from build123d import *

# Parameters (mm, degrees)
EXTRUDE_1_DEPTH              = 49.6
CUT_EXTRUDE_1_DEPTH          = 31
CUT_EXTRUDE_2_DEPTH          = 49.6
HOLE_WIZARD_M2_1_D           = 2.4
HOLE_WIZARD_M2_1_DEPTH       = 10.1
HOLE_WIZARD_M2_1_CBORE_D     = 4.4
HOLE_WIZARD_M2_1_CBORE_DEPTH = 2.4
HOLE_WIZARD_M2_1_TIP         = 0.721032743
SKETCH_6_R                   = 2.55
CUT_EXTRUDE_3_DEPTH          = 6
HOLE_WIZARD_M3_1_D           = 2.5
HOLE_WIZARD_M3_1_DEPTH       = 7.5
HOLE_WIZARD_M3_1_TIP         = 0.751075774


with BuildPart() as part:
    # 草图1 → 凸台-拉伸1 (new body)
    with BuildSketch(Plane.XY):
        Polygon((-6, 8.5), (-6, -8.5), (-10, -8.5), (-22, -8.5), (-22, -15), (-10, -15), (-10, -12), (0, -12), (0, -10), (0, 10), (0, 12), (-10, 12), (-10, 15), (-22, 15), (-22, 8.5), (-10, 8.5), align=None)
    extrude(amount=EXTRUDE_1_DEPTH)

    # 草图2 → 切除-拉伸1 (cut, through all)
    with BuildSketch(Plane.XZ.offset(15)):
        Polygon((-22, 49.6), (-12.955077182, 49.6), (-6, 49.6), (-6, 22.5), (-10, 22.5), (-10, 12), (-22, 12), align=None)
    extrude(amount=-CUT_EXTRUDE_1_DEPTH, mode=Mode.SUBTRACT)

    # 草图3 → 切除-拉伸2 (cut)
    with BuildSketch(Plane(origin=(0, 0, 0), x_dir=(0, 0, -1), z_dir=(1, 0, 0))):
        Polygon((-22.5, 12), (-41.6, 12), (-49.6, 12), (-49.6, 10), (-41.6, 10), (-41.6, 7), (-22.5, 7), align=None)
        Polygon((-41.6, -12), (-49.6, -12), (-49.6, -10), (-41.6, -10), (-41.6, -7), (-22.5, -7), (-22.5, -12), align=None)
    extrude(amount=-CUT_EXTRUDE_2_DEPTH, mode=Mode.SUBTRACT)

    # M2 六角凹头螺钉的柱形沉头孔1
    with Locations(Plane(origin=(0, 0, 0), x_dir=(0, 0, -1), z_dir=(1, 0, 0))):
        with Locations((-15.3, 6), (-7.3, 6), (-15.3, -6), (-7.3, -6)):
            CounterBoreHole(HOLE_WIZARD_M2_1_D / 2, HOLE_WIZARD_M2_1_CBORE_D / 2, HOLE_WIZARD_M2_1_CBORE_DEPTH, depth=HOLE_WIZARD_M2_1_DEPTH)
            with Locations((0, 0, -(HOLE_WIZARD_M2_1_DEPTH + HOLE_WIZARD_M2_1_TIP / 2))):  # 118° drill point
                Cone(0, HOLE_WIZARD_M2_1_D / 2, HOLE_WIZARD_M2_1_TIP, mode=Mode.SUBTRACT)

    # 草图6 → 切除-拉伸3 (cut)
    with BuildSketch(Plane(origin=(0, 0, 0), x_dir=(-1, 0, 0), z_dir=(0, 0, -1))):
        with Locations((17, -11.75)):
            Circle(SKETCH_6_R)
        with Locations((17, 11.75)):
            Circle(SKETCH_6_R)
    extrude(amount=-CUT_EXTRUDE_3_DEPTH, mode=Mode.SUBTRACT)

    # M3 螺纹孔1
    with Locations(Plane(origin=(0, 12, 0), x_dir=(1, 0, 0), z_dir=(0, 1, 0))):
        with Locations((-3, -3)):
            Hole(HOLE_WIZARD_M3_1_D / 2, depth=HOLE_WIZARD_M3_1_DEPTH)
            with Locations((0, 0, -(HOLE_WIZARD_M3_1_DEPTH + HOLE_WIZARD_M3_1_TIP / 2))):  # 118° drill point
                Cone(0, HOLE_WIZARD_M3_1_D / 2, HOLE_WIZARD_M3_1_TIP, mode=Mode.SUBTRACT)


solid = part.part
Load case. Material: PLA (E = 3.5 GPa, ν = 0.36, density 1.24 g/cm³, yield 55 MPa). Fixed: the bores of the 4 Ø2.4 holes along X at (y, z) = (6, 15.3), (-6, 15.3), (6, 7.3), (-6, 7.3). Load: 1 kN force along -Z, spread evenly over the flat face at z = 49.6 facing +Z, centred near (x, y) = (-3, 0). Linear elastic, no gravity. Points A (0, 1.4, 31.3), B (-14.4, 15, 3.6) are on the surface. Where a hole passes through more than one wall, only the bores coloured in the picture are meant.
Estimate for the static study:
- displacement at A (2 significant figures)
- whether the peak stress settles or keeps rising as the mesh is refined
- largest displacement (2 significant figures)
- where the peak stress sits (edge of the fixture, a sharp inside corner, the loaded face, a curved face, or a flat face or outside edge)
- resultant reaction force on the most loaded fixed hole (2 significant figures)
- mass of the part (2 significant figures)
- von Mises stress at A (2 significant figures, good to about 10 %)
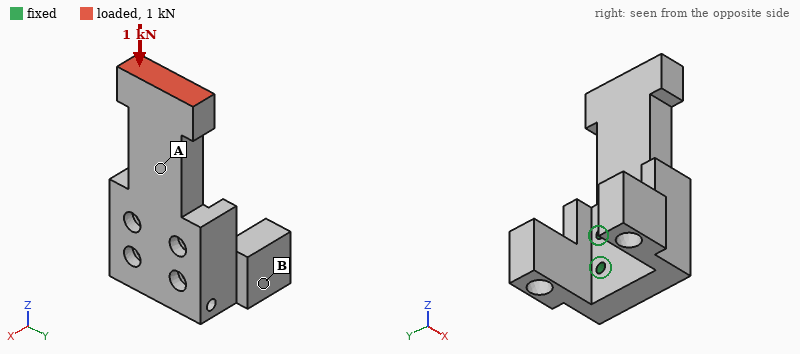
0.090 mm
keeps rising
0.18 mm
edge of the fixture
390 N
9.7 g
12 MPa
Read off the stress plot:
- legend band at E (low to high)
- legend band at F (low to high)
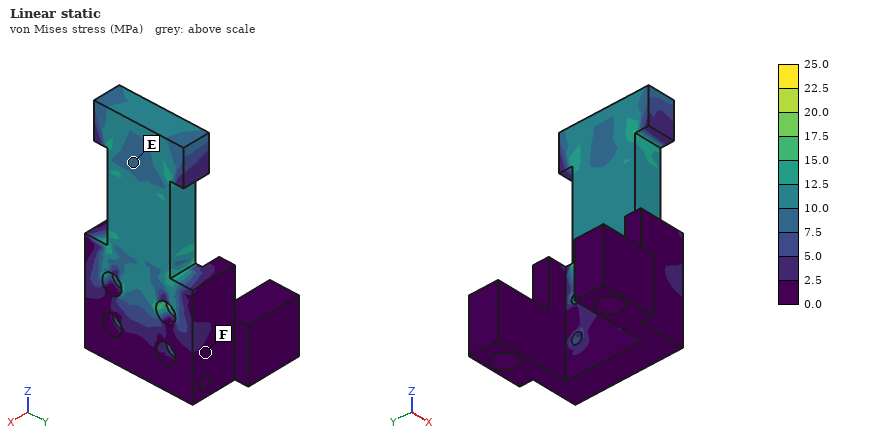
7.5 to 10.0 MPa
0.0 to 2.5 MPa
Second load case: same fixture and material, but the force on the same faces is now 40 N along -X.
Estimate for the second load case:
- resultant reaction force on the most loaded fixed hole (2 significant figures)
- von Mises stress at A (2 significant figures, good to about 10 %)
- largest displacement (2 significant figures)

78 N
8.7 MPa
0.62 mm
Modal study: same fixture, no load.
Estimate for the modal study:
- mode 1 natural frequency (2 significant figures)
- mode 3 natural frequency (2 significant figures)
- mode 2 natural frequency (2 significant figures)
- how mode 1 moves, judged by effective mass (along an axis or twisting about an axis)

1200 Hz
2400 Hz
2300 Hz
along X
